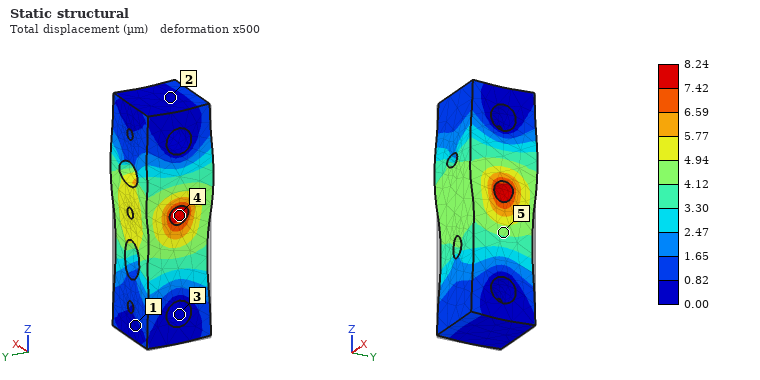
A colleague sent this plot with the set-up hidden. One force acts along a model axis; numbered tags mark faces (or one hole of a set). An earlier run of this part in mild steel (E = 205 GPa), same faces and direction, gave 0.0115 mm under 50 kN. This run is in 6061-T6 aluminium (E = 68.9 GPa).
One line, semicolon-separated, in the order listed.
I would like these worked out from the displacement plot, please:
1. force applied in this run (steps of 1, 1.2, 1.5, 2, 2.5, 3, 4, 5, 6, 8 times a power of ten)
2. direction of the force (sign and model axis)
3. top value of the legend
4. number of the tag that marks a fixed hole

12 kN; +Z; 8.24 µm; 3
